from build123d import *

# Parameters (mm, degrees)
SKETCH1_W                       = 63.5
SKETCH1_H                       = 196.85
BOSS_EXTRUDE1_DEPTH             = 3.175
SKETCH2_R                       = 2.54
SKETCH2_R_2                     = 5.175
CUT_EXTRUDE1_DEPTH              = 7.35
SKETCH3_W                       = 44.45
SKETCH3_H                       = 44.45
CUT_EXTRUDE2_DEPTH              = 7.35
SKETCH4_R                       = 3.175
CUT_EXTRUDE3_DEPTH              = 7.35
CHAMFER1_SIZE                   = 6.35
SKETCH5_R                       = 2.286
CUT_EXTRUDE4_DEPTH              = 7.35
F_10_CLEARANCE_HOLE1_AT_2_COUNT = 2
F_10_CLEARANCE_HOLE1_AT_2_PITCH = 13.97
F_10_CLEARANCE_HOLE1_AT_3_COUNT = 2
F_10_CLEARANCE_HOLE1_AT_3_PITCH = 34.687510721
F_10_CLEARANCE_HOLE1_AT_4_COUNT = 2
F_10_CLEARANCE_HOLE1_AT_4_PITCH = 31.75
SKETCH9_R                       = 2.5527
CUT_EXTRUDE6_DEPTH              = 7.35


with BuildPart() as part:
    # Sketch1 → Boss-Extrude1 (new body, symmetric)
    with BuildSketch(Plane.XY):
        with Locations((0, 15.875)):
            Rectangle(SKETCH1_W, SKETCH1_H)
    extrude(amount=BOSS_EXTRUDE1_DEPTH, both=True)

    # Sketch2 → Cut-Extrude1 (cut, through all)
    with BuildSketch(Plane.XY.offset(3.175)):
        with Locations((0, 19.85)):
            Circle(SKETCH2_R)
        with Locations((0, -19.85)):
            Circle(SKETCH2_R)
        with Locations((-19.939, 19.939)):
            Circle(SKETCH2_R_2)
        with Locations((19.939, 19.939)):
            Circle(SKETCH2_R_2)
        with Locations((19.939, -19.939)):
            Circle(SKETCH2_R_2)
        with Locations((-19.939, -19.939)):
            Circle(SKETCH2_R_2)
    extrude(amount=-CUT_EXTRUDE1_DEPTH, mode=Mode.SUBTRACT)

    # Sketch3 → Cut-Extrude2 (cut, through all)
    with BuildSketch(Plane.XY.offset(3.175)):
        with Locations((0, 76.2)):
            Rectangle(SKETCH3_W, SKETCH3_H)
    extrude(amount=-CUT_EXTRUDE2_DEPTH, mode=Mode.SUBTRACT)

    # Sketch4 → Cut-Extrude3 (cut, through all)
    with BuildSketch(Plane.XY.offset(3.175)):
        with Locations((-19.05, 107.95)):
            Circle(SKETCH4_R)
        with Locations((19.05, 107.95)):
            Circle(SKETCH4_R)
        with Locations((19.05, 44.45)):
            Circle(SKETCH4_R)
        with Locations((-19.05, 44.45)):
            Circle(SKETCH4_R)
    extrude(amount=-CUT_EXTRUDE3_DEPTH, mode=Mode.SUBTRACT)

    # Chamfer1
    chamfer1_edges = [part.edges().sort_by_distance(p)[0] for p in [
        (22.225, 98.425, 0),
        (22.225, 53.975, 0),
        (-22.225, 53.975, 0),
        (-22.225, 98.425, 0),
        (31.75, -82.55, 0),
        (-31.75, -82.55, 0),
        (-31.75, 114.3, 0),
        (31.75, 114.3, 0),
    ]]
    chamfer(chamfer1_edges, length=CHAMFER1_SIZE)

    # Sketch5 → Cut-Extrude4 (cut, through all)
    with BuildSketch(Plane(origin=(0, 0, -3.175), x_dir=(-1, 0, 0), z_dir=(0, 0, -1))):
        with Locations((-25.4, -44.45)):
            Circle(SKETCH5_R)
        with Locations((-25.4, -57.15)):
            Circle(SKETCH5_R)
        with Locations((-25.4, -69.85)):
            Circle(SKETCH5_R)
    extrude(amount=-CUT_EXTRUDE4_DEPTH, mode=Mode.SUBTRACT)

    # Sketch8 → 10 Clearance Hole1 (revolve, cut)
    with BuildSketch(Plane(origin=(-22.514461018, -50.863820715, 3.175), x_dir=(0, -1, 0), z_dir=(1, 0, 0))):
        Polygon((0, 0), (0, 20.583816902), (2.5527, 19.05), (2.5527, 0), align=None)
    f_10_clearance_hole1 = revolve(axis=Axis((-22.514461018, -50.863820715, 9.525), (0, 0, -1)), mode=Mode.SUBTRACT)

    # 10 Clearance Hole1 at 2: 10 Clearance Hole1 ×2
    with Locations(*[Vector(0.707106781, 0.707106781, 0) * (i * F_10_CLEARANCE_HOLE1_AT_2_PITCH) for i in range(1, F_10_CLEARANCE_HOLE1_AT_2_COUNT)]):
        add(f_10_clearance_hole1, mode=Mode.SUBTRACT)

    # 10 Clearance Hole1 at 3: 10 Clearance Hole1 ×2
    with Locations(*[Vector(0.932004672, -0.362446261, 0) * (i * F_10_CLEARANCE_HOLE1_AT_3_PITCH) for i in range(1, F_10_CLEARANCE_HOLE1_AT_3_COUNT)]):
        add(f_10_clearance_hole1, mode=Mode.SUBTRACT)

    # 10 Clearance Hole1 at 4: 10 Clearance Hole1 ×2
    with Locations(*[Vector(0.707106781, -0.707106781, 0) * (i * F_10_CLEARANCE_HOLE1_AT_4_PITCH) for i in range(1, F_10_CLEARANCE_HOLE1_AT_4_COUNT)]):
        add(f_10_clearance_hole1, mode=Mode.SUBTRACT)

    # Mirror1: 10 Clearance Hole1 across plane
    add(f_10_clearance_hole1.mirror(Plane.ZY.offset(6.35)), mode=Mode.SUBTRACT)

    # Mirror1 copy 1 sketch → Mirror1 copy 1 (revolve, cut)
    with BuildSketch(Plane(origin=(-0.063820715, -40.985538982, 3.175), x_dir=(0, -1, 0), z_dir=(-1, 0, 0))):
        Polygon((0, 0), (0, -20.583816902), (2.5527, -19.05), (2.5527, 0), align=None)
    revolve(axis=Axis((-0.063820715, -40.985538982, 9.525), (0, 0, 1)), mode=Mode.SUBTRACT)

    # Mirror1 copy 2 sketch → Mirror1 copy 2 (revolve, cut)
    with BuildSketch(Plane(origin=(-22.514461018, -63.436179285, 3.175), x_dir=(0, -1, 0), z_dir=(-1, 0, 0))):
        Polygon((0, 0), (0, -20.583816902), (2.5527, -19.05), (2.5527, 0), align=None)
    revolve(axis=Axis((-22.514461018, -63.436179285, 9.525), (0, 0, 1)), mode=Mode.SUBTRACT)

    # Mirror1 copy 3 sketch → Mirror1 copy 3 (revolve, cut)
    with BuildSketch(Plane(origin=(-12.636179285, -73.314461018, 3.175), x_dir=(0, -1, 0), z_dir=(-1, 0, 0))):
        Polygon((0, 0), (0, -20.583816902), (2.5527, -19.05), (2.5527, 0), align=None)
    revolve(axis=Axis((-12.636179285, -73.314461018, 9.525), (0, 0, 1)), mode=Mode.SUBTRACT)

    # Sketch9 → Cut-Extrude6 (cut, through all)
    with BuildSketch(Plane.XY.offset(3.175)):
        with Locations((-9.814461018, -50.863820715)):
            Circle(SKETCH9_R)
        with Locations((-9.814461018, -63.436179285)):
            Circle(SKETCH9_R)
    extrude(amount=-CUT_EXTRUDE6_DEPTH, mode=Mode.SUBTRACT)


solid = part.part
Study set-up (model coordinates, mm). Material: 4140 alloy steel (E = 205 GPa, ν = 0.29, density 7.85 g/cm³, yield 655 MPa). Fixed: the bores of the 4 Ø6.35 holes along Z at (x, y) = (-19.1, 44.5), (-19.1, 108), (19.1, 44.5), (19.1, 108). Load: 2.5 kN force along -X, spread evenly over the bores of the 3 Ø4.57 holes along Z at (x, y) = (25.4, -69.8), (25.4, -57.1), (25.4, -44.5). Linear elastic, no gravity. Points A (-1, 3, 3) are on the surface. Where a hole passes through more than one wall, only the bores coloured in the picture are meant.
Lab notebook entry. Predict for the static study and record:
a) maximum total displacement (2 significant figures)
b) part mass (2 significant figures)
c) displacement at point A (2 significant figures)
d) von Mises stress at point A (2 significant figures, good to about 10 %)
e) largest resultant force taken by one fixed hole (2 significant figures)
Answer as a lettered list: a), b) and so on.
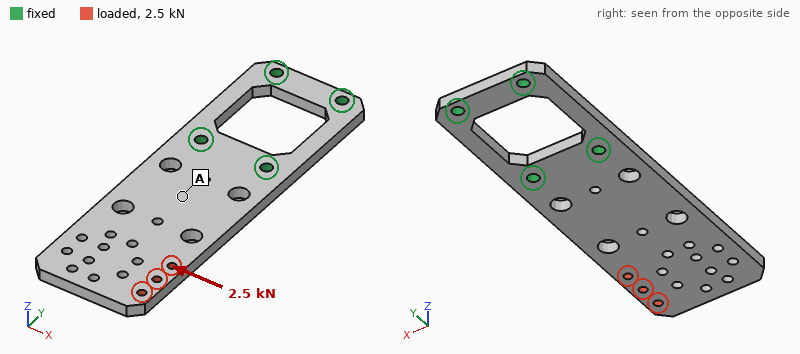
a) 75 µm
b) 490 g
c) 15 µm
d) 17 MPa
e) 5.7 kN
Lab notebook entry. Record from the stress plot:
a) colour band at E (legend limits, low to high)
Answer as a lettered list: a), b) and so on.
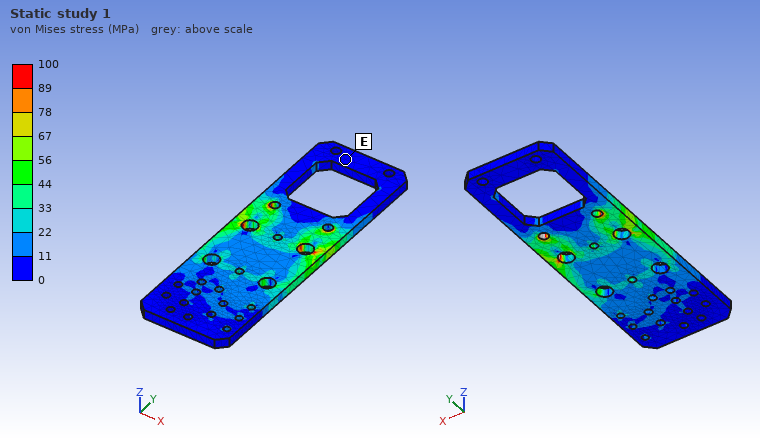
a) 0 to 11 MPa
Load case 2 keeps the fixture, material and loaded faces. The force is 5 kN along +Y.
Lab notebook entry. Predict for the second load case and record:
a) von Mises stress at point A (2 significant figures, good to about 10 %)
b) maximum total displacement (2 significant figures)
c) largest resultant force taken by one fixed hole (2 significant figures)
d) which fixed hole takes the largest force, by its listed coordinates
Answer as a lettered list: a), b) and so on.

a) 13 MPa
b) 54 µm
c) 5.2 kN
d) (19.1, 44.5)
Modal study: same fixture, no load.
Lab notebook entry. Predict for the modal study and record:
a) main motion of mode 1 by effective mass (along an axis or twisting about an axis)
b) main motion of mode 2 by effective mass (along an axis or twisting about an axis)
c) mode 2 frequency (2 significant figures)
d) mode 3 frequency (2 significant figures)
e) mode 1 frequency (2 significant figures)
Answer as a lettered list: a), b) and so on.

a) along Z
b) twisting about Y
c) 1400 Hz
d) 2000 Hz
e) 320 Hz
